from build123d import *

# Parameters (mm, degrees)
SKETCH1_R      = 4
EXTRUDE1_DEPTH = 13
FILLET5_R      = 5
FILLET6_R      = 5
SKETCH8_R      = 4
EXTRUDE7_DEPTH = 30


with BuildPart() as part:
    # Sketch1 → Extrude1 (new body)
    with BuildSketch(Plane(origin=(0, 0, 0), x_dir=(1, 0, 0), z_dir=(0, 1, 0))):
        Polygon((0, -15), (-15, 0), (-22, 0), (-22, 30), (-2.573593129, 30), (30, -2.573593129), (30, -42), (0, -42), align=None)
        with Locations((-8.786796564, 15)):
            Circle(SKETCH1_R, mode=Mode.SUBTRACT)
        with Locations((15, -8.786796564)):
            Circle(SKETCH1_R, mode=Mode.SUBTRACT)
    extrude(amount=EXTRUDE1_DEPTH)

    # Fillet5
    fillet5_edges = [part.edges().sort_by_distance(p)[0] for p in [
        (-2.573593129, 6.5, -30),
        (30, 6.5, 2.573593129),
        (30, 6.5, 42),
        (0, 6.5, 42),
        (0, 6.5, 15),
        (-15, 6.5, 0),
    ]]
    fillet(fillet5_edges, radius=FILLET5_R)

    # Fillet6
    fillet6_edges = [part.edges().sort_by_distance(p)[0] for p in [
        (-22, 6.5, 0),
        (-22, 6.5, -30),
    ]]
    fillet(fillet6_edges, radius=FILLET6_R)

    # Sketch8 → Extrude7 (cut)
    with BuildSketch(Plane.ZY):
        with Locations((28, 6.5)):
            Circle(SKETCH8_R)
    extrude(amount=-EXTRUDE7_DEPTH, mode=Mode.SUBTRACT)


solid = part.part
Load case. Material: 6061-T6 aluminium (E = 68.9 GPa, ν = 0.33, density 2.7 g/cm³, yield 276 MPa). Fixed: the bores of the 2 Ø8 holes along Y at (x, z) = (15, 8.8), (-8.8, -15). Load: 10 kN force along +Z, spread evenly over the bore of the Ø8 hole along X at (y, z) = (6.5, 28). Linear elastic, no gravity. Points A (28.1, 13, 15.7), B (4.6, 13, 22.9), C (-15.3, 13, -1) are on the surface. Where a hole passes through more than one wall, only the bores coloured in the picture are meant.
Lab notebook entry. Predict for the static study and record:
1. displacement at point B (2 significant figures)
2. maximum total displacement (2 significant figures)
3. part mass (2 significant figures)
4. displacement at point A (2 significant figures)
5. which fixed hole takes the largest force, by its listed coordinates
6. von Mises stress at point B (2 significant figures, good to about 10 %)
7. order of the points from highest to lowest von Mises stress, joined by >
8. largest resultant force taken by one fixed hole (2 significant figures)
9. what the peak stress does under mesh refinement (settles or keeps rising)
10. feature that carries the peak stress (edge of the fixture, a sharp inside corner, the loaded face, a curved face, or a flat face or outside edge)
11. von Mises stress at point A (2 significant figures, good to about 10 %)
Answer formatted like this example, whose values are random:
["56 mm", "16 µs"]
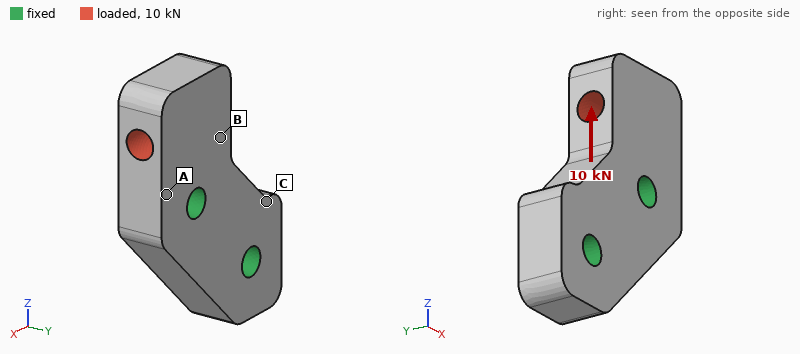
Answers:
["6.3 µm", "15 µm", "76 g", "7.2 µm", "(15, 8.8)", "34 MPa", "B > A > C", "9.0 kN", "keeps rising", "edge of the fixture", "19 MPa"]
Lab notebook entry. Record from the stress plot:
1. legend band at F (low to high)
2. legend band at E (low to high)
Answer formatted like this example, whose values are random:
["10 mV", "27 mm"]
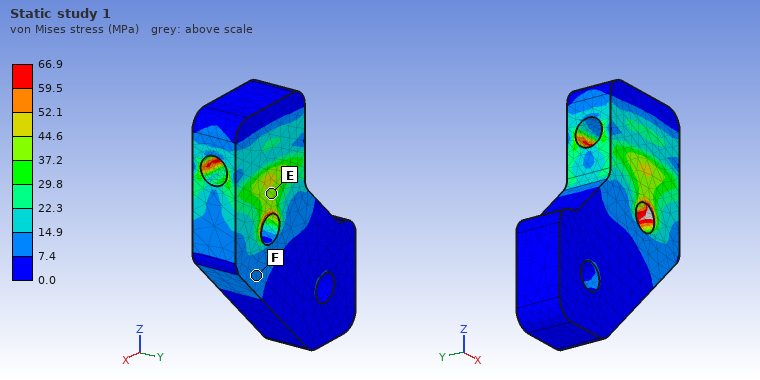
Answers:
["7.4 to 14.9 MPa", "37.2 to 44.6 MPa"]
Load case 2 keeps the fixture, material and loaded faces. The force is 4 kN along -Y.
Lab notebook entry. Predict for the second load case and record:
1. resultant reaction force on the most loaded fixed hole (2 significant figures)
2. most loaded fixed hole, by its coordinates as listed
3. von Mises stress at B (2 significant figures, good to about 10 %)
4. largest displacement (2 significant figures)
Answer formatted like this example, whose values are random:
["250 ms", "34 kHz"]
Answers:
["4.4 kN", "(15, 8.8)", "47 MPa", "71 µm"]
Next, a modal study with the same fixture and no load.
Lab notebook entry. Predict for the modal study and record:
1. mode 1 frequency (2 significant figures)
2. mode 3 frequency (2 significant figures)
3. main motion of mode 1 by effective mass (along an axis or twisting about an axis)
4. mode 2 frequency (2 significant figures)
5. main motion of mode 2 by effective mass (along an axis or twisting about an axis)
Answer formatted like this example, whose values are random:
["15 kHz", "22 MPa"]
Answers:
["8600 Hz", "16 kHz", "along Y", "13 kHz", "along X"]
